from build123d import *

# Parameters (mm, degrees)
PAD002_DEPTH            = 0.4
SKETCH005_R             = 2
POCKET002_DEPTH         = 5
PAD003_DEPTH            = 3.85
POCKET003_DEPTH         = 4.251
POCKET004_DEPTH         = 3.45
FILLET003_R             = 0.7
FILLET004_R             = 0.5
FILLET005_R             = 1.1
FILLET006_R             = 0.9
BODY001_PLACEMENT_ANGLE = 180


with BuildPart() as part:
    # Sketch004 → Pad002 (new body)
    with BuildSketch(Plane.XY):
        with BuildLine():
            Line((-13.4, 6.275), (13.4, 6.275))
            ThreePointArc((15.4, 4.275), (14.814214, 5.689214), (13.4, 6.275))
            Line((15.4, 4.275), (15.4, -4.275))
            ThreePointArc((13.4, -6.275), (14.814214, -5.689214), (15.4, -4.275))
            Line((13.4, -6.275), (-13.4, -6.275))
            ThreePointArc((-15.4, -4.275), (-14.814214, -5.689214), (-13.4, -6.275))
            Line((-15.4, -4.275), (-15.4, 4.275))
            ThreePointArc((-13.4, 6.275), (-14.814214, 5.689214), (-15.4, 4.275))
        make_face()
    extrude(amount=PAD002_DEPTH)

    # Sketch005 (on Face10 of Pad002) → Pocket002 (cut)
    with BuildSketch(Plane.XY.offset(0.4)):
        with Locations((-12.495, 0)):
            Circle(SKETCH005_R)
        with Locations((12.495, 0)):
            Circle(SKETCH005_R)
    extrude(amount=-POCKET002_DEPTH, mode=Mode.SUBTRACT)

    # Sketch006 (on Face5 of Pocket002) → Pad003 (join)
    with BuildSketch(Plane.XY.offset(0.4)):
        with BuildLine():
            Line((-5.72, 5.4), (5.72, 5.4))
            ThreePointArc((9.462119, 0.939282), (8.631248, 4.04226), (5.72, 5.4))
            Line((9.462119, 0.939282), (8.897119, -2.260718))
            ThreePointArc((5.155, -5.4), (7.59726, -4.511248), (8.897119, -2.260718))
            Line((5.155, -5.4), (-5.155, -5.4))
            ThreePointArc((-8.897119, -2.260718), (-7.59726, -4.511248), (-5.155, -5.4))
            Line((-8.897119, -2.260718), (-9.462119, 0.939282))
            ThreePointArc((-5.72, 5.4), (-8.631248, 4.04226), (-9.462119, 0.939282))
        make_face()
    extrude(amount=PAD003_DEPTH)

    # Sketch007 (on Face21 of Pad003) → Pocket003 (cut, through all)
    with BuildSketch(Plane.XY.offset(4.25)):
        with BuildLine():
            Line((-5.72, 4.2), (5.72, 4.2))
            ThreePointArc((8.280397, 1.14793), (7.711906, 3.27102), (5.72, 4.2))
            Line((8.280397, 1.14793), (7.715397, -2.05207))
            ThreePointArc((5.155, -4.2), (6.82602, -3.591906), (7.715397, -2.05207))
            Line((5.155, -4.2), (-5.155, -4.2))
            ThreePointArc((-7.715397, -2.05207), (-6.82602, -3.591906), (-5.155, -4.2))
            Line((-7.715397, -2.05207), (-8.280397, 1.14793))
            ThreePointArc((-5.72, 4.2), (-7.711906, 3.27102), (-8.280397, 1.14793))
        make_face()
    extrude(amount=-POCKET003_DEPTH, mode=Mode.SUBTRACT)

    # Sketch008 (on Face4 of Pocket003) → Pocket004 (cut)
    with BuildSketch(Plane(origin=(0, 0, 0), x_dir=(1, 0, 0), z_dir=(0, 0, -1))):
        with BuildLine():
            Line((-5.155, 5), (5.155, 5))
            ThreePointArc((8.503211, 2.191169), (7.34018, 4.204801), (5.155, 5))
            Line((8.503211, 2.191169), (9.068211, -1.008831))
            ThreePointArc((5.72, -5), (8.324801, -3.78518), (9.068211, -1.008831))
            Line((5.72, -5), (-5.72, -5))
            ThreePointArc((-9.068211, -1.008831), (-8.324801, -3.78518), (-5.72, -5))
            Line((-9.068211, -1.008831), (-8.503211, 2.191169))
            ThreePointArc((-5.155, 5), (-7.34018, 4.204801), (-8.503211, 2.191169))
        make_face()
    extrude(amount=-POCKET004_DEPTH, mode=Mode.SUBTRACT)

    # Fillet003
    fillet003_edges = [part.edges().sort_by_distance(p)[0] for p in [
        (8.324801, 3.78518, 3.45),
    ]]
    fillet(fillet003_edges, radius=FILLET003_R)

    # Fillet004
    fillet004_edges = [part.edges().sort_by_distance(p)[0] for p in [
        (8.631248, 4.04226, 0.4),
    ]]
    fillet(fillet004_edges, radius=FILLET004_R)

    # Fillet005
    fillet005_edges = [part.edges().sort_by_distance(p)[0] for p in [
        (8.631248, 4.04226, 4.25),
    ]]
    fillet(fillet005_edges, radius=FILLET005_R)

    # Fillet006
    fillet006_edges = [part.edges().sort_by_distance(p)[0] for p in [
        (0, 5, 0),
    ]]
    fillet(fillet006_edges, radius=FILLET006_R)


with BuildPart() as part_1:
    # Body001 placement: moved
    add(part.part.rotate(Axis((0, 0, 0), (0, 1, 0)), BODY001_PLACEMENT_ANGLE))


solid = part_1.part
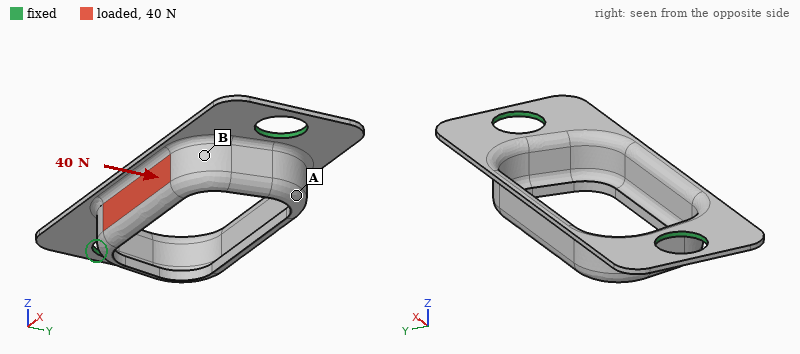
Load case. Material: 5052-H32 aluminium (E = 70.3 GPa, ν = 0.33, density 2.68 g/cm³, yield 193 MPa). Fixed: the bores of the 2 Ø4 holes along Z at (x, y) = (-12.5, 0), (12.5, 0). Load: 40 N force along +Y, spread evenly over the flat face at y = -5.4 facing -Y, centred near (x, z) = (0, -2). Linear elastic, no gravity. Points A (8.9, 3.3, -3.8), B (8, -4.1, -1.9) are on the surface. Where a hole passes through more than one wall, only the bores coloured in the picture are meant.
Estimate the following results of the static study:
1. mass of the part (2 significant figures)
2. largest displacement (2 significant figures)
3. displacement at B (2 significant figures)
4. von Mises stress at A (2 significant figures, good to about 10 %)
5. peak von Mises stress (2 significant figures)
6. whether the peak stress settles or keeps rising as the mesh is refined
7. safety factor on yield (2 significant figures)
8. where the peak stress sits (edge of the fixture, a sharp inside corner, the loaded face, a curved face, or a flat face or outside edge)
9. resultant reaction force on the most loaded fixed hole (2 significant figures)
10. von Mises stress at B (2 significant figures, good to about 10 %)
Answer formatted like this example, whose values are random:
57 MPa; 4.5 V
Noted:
0.46 g; 79 µm; 26 µm; 25 MPa; 170 MPa; settles; 1.1; a flat face or outside edge; 27 N; 45 MPa
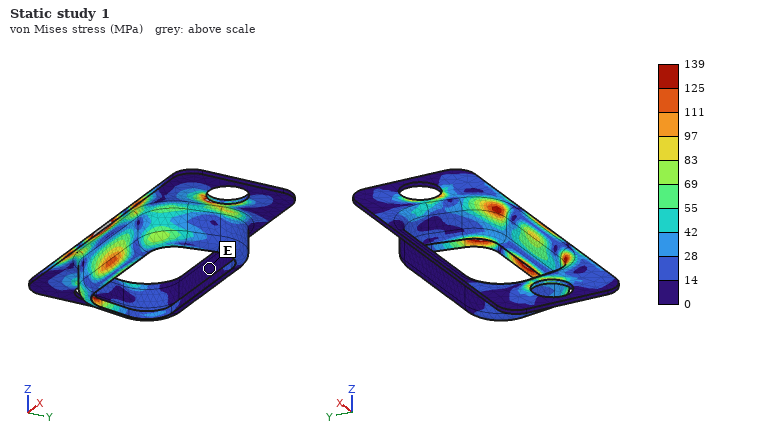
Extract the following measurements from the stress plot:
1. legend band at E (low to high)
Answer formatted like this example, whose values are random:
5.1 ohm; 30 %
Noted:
0 to 14 MPa
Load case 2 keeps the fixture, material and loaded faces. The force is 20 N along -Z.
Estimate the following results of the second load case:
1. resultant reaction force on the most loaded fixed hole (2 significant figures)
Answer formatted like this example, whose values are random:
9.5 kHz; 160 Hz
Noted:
16 N
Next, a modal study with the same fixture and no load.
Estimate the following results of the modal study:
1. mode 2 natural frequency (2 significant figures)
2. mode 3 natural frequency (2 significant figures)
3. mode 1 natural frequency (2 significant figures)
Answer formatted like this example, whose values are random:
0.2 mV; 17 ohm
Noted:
14 kHz; 14 kHz; 7200 Hz
